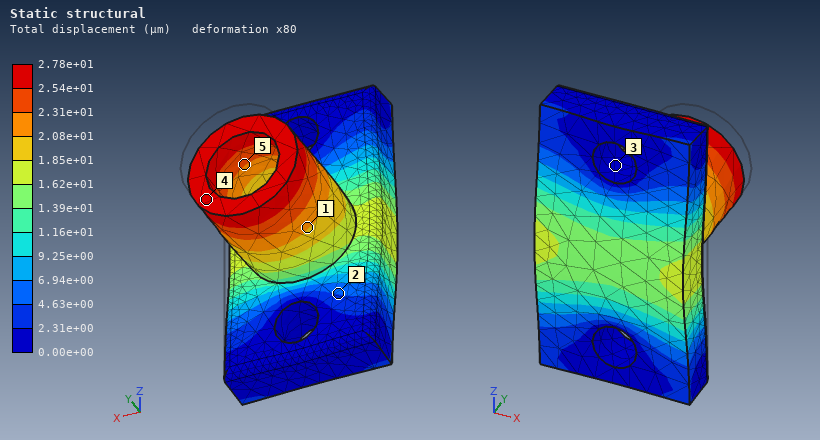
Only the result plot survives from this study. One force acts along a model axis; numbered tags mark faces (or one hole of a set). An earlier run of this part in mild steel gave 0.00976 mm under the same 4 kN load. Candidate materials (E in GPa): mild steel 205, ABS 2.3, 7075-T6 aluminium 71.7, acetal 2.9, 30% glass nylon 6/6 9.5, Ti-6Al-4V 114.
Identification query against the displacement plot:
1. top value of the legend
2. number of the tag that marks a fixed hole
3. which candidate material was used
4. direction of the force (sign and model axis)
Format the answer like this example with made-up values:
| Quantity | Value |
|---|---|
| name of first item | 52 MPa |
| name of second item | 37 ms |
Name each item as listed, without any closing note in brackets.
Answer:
| Quantity | Value |
|---|---|
| top value of the legend | 2.78e+01 µm |
| number of the tag that marks a fixed hole | 3 |
| which candidate material was used | 7075-T6 aluminium |
| direction of the force | -Y |
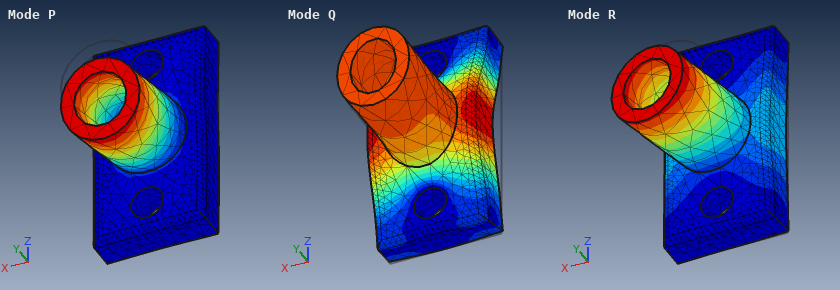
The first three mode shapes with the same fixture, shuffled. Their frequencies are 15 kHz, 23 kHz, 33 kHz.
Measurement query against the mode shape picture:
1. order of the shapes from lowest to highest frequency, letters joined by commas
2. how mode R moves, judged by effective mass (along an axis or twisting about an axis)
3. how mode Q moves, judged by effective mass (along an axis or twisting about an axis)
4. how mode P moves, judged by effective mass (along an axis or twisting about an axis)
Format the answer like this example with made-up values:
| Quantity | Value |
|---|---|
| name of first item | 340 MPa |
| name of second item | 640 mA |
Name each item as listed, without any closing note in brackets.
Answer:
| Quantity | Value |
|---|---|
| order of the shapes from lowest to highest frequency, letters joined by commas | R, P, Q |
| how mode R moves, judged by effective mass | along X |
| how mode Q moves, judged by effective mass | along Y |
| how mode P moves, judged by effective mass | along Z |
